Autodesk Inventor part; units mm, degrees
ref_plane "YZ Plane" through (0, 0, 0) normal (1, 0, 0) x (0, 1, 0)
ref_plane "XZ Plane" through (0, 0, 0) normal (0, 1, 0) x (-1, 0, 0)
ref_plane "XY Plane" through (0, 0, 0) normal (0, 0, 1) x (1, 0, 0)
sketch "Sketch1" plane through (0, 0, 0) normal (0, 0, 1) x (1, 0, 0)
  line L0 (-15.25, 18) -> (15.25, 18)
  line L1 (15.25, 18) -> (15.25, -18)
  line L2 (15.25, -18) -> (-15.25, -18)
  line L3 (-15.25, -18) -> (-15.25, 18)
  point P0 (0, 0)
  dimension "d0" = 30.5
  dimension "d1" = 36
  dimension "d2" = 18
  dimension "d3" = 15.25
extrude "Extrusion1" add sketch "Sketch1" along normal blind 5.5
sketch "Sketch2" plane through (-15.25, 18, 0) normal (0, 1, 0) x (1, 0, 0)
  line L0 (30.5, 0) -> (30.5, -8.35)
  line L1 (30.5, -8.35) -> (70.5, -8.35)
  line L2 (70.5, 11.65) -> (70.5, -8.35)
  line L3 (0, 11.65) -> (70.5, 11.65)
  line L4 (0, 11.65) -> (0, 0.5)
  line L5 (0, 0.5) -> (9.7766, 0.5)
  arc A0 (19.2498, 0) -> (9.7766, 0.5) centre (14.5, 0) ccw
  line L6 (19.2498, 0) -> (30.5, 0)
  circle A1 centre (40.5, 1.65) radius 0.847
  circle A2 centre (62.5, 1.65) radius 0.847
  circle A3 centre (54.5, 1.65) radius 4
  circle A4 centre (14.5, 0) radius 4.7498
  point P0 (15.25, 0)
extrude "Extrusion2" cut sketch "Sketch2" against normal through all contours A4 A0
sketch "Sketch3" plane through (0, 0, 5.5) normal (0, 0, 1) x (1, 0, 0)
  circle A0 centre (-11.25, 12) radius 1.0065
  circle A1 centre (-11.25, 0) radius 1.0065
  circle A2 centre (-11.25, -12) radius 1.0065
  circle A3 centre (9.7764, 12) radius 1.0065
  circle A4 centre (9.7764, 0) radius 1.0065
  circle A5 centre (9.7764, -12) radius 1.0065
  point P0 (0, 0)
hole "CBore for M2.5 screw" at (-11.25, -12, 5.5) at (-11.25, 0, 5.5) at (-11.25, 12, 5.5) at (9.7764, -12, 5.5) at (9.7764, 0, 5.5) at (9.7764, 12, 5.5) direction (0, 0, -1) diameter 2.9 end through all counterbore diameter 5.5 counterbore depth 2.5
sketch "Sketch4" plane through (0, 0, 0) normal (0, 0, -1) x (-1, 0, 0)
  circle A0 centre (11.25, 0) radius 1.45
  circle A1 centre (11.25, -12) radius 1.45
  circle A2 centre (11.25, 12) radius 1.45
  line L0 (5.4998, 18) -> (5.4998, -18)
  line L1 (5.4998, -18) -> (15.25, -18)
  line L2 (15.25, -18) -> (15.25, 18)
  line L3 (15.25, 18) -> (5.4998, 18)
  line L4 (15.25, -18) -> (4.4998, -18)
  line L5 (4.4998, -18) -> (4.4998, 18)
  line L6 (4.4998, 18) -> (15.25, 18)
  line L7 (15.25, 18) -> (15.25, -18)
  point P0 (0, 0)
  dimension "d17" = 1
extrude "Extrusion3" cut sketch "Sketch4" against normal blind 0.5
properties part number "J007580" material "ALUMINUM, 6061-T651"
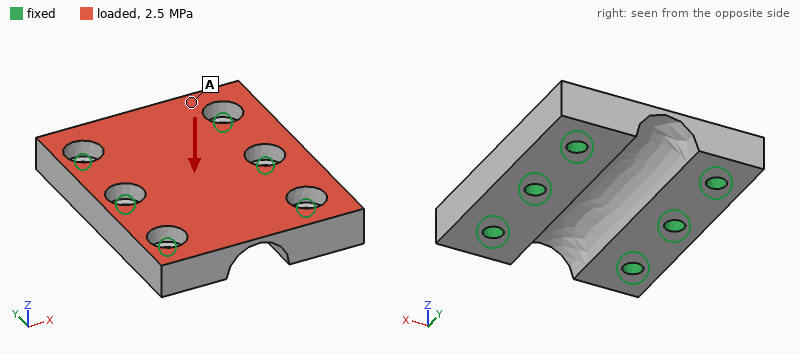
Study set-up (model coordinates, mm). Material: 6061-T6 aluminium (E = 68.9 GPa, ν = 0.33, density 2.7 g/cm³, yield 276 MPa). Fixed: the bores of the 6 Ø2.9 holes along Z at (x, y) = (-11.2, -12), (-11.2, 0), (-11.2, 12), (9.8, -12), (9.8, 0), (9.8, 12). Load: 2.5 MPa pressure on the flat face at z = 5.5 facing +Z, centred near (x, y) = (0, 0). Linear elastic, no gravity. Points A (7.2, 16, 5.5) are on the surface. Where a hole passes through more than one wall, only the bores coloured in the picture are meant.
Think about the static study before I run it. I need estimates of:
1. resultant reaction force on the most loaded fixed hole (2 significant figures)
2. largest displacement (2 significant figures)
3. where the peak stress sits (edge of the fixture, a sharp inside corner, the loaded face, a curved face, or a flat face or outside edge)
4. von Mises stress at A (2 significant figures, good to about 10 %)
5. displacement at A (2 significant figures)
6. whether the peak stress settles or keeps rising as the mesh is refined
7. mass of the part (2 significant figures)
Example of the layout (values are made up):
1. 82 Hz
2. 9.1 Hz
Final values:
1. 510 N
2. 8.0 µm
3. edge of the fixture
4. 7.9 MPa
5. 2.7 µm
6. keeps rising
7. 11 g
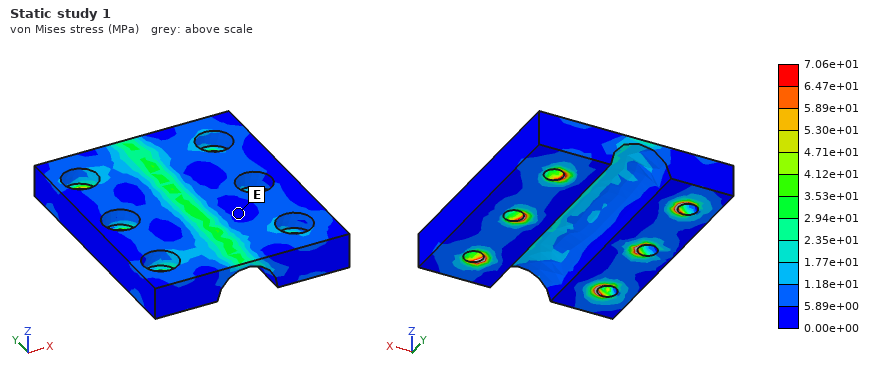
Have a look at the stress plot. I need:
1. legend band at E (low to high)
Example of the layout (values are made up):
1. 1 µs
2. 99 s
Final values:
1. 0.00e+00 to 5.89e+00 MPa
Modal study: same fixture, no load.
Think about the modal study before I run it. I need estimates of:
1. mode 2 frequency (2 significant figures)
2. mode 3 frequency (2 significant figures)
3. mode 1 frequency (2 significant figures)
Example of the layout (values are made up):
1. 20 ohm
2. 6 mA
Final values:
1. 43 kHz
2. 44 kHz
3. 42 kHz
